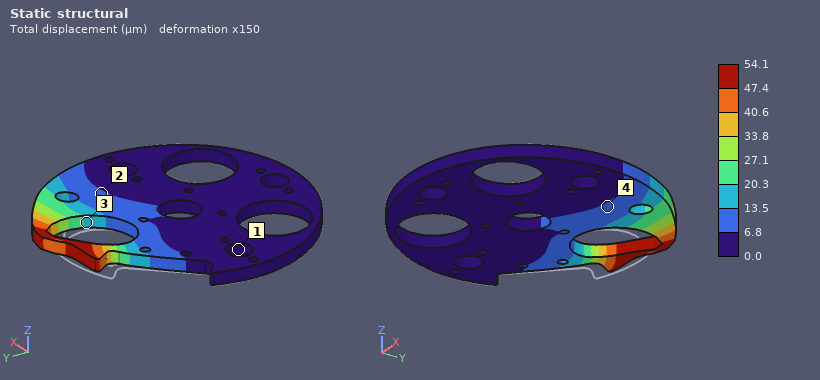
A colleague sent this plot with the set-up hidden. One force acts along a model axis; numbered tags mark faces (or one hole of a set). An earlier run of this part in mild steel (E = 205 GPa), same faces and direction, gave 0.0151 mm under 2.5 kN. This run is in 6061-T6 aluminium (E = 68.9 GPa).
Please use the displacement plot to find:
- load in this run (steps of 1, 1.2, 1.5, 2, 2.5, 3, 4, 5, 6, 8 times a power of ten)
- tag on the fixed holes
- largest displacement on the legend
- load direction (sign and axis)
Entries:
3 kN
1
54.1 µm
+X
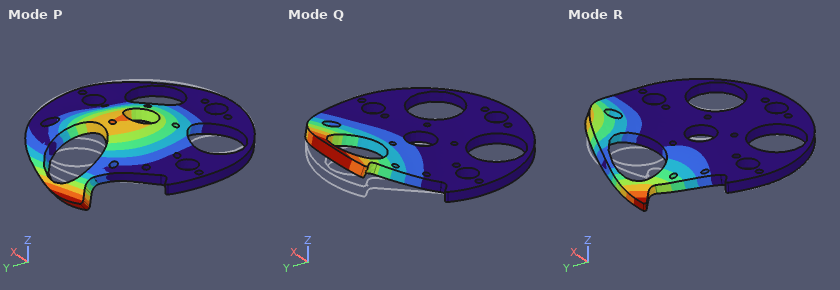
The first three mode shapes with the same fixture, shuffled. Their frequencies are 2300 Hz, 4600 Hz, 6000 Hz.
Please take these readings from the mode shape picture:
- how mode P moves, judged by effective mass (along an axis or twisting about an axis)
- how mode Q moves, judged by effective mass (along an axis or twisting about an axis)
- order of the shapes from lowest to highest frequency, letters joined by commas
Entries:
along Z
along Z
Q, R, P
